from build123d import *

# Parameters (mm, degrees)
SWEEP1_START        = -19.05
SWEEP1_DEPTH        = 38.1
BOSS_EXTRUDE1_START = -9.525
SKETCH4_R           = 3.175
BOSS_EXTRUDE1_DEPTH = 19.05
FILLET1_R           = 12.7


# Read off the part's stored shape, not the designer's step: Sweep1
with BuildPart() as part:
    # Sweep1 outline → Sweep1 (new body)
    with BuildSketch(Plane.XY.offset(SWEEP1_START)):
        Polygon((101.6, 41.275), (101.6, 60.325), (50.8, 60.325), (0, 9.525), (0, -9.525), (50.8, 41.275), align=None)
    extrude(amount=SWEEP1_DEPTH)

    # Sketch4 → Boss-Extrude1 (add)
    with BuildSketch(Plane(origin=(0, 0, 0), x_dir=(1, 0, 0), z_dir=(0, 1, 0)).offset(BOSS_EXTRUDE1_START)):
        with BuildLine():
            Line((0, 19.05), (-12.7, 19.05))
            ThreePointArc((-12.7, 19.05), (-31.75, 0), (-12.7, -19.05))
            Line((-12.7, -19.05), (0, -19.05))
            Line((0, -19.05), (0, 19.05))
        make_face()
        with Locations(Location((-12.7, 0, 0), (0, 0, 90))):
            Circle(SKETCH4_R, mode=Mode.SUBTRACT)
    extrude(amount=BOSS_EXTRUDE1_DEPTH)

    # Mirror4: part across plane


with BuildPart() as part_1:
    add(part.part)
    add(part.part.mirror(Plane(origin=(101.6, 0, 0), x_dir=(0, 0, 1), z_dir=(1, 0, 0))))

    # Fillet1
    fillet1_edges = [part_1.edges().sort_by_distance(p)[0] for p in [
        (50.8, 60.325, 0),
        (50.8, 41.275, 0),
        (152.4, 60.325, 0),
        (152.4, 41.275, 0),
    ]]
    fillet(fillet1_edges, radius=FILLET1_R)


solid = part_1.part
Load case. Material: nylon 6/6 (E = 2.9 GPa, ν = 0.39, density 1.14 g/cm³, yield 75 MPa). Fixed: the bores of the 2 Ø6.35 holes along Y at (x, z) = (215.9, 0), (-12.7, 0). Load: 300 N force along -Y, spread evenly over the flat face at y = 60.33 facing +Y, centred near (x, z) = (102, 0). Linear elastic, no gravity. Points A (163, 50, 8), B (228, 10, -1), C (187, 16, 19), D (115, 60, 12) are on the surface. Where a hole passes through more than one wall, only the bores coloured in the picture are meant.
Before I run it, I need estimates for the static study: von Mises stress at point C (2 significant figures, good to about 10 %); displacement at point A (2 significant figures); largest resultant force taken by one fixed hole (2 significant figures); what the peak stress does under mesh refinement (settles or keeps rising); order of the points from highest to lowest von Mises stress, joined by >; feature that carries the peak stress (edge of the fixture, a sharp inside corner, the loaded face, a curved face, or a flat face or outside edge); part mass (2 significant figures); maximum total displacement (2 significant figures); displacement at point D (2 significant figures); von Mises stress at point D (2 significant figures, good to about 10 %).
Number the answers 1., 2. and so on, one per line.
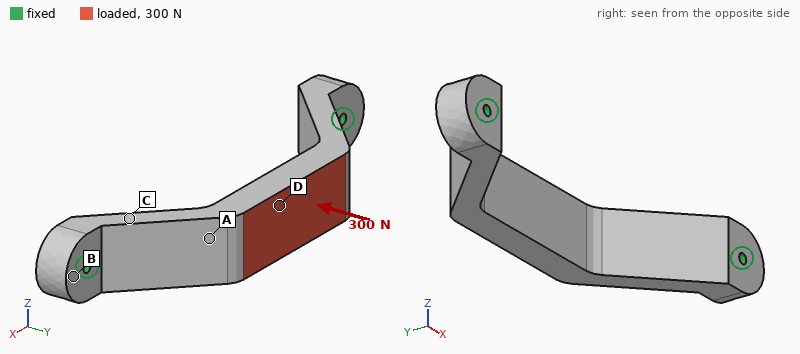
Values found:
1. 0.51 MPa
2. 16 µm
3. 240 N
4. keeps rising
5. D > C > A > B
6. edge of the fixture
7. 210 g
8. 76 µm
9. 70 µm
10. 1.3 MPa
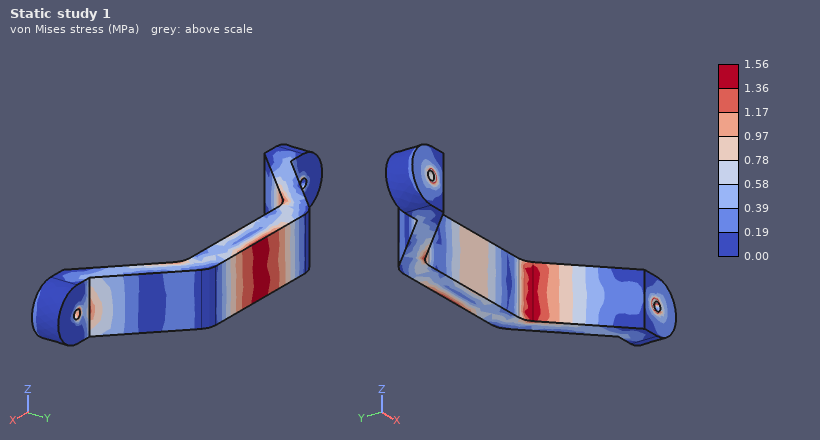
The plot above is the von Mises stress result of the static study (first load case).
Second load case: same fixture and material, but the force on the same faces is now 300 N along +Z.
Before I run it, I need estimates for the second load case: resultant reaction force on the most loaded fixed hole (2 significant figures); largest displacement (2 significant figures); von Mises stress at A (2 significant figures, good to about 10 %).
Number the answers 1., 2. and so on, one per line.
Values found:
1. 150 N
2. 0.59 mm
3. 2.0 MPa
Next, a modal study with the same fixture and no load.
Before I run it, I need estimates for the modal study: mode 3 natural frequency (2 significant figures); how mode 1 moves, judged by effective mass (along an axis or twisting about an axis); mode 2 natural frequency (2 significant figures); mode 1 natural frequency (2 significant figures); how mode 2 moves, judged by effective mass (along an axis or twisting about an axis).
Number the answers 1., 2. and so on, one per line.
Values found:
1. 1100 Hz
2. along Z
3. 780 Hz
4. 400 Hz
5. along X
